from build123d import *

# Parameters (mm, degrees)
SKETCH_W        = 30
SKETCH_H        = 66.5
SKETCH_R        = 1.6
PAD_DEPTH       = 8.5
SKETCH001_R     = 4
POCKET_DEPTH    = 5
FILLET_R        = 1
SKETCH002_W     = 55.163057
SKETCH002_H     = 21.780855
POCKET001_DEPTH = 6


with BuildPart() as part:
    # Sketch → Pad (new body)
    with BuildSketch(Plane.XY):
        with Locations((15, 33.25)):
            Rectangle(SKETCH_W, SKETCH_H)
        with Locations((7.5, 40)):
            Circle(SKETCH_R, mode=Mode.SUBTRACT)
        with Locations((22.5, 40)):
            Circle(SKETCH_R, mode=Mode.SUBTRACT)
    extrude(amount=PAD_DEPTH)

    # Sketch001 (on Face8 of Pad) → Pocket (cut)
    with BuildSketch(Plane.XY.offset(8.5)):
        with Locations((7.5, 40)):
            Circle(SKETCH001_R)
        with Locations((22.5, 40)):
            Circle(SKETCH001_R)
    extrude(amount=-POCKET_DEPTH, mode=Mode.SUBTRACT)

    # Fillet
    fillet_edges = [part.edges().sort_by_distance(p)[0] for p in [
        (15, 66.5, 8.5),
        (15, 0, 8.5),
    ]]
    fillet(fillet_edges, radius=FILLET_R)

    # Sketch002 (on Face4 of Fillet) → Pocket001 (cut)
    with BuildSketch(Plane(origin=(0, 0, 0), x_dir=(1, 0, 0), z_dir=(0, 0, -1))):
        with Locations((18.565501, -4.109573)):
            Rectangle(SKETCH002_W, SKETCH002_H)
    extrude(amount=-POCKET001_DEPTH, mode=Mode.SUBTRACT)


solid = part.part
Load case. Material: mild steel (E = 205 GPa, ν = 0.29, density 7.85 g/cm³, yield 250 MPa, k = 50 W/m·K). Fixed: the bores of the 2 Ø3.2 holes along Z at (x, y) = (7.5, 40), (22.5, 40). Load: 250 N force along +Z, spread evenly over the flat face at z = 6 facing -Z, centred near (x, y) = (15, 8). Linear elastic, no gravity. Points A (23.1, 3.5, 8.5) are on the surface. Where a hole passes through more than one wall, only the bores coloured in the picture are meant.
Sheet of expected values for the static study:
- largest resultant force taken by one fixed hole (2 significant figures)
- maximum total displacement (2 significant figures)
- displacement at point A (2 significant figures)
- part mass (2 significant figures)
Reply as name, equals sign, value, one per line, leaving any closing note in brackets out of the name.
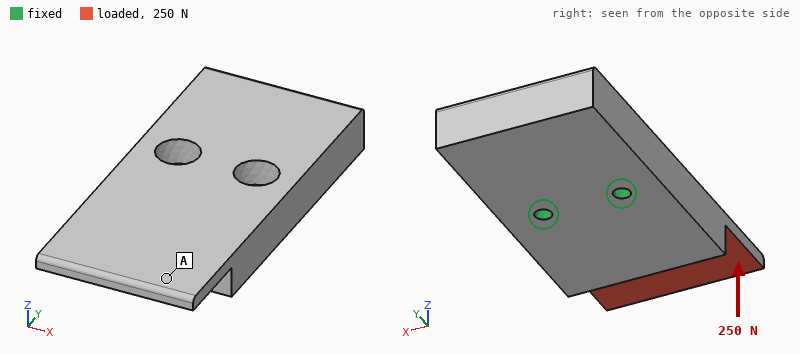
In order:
largest resultant force taken by one fixed hole = 130 N
maximum total displacement = 54 µm
displacement at point A = 46 µm
part mass = 110 g
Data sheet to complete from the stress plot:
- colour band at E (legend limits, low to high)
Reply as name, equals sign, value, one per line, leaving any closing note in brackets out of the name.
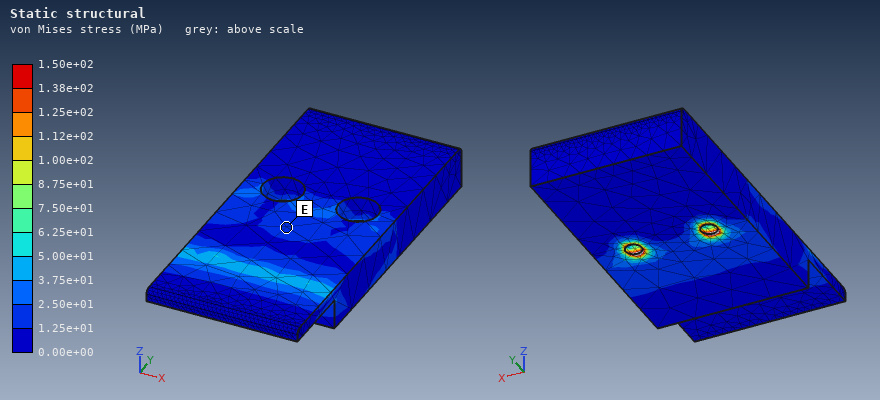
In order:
colour band at E = 1.25e+01 to 2.50e+01 MPa
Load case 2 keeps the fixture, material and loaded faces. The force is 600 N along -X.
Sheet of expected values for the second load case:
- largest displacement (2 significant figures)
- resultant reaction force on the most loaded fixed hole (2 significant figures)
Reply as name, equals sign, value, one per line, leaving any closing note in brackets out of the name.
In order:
largest displacement = 11 µm
resultant reaction force on the most loaded fixed hole = 1.2 kN
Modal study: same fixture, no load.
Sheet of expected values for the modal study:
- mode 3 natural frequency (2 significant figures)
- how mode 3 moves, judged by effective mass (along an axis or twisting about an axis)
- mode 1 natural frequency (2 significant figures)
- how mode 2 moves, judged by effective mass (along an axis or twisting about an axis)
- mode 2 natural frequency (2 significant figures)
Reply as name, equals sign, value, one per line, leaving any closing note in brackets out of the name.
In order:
mode 3 natural frequency = 9700 Hz
how mode 3 moves, judged by effective mass = twisting about Z
mode 1 natural frequency = 3000 Hz
how mode 2 moves, judged by effective mass = along Z
mode 2 natural frequency = 6700 Hz
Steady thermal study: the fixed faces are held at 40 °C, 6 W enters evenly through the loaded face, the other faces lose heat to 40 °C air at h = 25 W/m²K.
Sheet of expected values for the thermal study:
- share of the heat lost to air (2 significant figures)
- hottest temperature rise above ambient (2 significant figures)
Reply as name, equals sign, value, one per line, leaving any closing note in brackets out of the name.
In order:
share of the heat lost to air = 15 %
hottest temperature rise above ambient = 26 K
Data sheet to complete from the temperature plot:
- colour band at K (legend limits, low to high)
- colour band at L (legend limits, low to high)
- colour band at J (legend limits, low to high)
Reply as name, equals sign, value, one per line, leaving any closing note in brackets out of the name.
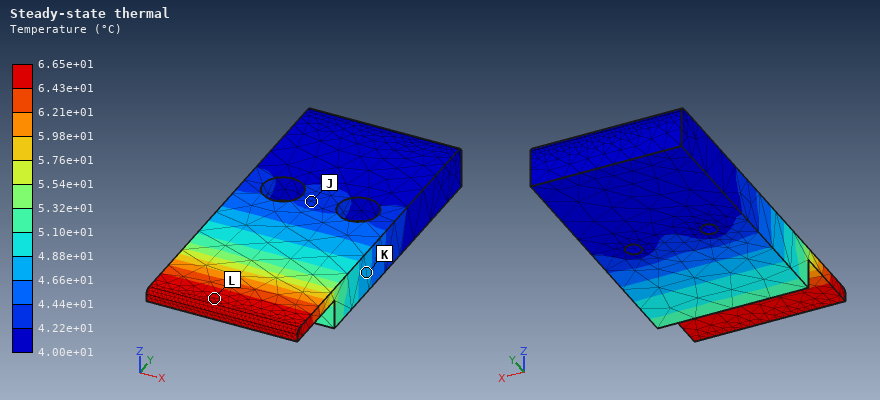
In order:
colour band at K = 4.66e+01 to 4.88e+01 °C
colour band at L = 6.43e+01 to 6.65e+01 °C
colour band at J = 4.22e+01 to 4.44e+01 °C
